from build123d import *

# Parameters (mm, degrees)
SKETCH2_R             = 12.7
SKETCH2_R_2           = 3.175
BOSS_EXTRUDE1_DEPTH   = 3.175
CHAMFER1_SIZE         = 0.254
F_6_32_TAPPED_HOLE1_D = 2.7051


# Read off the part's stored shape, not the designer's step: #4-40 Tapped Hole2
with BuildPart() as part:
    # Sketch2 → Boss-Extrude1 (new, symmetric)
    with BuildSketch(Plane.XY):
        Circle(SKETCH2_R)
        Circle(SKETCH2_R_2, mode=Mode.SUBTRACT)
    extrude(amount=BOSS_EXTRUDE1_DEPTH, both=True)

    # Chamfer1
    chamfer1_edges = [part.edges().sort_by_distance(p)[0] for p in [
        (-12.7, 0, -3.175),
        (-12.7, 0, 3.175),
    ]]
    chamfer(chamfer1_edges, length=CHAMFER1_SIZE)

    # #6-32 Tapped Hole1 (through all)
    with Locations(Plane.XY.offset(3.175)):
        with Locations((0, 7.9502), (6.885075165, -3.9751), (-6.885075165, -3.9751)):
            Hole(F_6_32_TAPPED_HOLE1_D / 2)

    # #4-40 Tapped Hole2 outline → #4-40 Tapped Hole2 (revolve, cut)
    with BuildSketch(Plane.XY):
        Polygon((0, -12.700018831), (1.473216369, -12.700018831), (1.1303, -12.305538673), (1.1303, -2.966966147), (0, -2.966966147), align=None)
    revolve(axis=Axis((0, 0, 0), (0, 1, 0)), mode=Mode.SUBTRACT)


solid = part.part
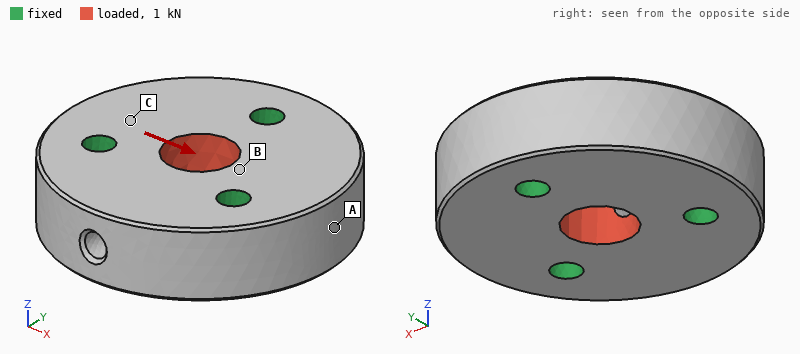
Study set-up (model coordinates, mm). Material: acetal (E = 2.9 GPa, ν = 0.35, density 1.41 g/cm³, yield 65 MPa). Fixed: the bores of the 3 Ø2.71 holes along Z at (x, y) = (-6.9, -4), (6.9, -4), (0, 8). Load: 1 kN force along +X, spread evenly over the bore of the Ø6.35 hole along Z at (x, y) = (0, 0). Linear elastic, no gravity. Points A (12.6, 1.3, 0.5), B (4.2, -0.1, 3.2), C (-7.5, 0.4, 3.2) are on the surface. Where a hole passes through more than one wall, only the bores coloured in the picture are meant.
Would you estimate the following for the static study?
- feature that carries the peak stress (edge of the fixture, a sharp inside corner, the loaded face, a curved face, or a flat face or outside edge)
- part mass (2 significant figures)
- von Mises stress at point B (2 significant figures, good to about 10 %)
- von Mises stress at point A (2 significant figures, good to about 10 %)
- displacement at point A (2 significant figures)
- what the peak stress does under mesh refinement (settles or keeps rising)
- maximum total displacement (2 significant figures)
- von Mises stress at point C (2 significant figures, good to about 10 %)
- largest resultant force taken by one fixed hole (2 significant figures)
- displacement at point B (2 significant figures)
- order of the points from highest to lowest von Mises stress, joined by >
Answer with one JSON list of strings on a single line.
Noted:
["edge of the fixture", "4.0 g", "8.2 MPa", "2.6 MPa", "9.4 µm", "keeps rising", "25 µm", "5.5 MPa", "350 N", "18 µm", "B > C > A"]
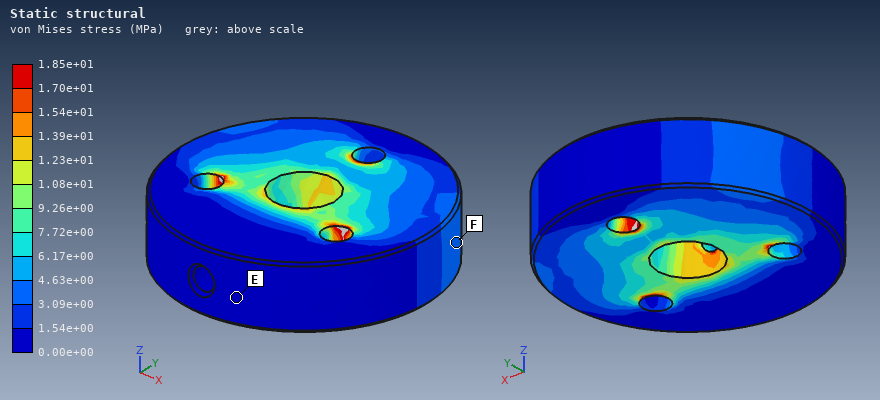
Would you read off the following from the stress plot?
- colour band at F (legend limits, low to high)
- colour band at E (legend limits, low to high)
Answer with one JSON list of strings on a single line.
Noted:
["3.09e+00 to 4.63e+00 MPa", "0.00e+00 to 1.54e+00 MPa"]
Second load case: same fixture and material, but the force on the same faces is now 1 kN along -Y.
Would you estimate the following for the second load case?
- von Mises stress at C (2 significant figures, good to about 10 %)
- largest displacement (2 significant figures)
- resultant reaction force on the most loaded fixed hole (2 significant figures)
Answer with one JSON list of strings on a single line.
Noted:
["3.2 MPa", "27 µm", "340 N"]
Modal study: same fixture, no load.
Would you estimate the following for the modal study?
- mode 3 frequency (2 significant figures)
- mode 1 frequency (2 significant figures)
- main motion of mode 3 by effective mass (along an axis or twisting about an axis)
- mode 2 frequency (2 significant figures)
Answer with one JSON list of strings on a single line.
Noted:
["17 kHz", "15 kHz", "along Z", "15 kHz"]
